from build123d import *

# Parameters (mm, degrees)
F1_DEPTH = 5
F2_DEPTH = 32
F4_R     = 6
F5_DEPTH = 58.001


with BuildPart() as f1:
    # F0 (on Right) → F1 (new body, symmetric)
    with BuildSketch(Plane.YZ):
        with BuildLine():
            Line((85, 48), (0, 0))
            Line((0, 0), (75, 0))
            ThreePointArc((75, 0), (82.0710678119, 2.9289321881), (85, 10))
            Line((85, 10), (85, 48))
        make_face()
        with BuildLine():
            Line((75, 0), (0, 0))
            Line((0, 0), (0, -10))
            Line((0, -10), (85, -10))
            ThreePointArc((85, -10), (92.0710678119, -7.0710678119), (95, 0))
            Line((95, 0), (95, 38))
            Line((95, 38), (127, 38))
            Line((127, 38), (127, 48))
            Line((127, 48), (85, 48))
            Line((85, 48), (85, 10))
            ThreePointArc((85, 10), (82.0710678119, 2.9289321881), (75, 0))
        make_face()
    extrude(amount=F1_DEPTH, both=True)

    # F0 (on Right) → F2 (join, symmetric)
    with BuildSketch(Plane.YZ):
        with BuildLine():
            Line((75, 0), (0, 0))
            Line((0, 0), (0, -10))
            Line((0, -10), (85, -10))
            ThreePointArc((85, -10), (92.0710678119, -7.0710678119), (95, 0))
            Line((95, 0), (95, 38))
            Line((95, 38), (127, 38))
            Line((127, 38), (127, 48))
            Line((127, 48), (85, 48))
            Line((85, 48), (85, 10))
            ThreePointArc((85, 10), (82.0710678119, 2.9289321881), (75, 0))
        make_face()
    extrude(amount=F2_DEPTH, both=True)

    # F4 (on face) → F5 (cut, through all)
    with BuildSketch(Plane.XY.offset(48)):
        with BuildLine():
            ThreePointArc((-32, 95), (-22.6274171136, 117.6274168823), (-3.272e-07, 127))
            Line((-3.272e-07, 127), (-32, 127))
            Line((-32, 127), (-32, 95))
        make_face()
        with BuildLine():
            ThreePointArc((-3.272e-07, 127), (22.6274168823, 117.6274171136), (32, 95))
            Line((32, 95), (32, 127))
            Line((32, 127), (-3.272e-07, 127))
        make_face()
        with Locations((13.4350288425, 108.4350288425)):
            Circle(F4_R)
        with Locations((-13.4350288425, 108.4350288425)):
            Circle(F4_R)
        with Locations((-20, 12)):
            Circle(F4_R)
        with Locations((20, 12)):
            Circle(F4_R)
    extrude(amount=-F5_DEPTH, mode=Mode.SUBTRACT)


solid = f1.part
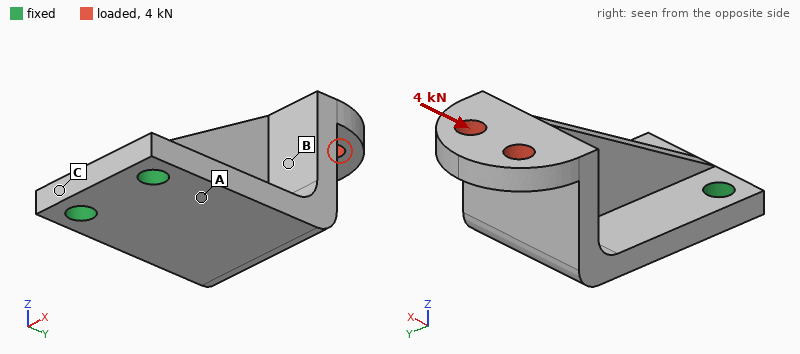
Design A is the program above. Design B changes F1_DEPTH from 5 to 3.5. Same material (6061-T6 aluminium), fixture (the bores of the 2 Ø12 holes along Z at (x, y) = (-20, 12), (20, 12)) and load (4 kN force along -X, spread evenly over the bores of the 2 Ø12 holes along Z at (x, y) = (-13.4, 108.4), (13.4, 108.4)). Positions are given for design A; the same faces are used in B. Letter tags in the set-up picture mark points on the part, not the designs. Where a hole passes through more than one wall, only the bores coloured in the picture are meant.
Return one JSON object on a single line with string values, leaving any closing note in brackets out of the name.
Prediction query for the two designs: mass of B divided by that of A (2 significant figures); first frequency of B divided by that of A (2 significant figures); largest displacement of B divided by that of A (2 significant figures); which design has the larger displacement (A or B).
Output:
{"mass of B divided by that of A": "0.95", "first frequency of B divided by that of A": "0.96", "largest displacement of B divided by that of A": "1.2", "which design has the larger displacement": "B"}
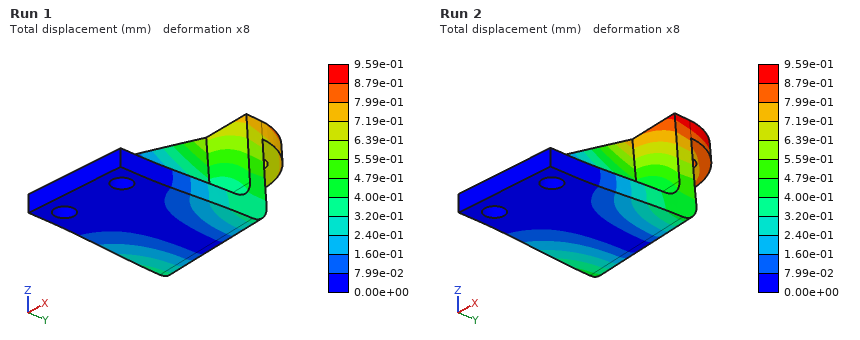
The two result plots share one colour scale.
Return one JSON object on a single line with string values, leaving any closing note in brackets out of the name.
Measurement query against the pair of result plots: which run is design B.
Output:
{"which run is design B": "Run 2"}
